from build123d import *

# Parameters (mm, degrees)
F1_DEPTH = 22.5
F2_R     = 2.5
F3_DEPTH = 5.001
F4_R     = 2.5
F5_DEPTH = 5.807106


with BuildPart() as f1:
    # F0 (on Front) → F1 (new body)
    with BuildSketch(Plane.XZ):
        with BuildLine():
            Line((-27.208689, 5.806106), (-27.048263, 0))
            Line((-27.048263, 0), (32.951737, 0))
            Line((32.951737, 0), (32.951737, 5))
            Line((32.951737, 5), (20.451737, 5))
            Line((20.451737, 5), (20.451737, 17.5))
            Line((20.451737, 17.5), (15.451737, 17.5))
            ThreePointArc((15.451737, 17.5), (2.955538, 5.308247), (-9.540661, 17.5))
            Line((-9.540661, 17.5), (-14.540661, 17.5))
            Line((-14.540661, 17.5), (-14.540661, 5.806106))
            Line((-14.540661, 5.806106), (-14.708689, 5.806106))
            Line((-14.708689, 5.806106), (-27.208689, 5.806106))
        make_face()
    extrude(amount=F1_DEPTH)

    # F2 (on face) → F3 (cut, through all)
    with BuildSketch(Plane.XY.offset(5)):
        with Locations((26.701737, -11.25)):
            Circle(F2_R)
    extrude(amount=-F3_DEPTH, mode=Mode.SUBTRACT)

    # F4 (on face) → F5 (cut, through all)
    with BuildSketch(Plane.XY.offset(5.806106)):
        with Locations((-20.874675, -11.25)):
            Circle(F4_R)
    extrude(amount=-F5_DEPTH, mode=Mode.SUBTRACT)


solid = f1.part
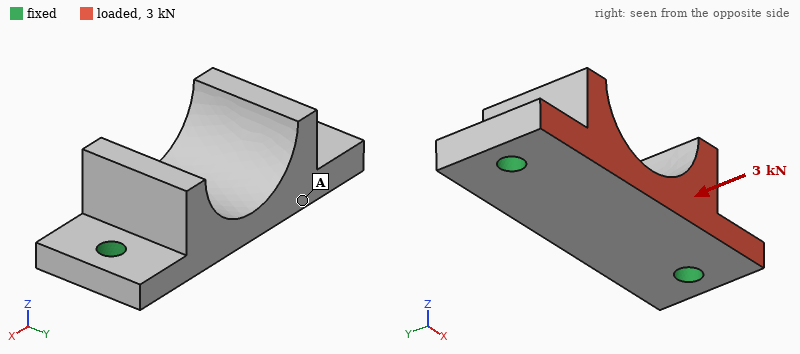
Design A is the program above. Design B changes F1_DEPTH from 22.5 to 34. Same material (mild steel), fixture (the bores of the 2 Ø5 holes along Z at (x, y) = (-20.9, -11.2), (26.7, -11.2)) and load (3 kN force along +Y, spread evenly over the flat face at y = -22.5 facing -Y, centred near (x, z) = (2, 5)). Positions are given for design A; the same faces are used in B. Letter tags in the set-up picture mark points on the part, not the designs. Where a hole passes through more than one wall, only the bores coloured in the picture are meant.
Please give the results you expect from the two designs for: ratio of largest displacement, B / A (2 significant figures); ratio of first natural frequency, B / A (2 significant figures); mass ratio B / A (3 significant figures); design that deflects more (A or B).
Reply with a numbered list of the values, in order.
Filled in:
1. 1.1
2. 0.60
3. 1.52
4. B
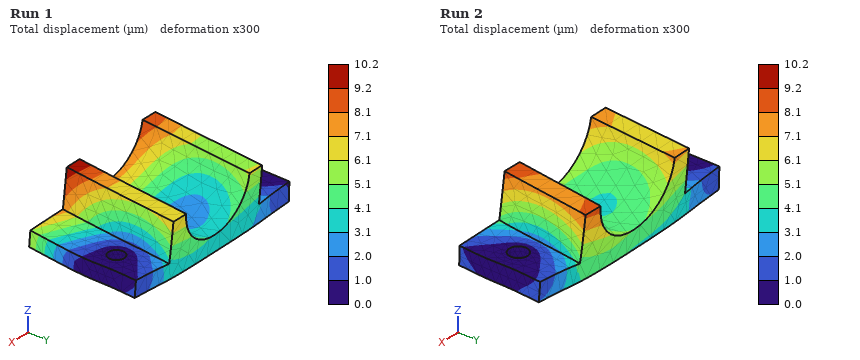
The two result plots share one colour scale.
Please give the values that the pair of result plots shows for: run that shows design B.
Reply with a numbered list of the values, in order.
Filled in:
1. Run 1
